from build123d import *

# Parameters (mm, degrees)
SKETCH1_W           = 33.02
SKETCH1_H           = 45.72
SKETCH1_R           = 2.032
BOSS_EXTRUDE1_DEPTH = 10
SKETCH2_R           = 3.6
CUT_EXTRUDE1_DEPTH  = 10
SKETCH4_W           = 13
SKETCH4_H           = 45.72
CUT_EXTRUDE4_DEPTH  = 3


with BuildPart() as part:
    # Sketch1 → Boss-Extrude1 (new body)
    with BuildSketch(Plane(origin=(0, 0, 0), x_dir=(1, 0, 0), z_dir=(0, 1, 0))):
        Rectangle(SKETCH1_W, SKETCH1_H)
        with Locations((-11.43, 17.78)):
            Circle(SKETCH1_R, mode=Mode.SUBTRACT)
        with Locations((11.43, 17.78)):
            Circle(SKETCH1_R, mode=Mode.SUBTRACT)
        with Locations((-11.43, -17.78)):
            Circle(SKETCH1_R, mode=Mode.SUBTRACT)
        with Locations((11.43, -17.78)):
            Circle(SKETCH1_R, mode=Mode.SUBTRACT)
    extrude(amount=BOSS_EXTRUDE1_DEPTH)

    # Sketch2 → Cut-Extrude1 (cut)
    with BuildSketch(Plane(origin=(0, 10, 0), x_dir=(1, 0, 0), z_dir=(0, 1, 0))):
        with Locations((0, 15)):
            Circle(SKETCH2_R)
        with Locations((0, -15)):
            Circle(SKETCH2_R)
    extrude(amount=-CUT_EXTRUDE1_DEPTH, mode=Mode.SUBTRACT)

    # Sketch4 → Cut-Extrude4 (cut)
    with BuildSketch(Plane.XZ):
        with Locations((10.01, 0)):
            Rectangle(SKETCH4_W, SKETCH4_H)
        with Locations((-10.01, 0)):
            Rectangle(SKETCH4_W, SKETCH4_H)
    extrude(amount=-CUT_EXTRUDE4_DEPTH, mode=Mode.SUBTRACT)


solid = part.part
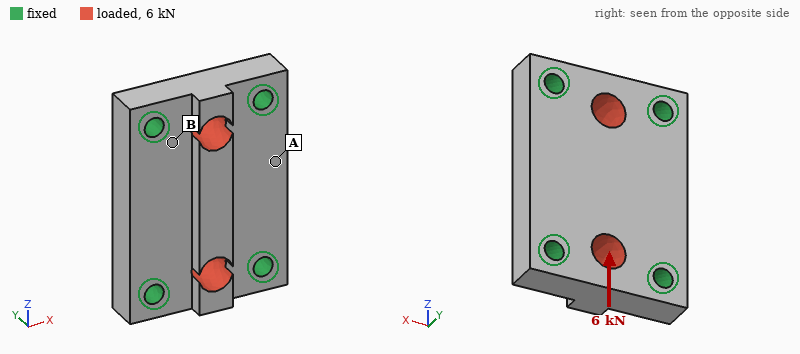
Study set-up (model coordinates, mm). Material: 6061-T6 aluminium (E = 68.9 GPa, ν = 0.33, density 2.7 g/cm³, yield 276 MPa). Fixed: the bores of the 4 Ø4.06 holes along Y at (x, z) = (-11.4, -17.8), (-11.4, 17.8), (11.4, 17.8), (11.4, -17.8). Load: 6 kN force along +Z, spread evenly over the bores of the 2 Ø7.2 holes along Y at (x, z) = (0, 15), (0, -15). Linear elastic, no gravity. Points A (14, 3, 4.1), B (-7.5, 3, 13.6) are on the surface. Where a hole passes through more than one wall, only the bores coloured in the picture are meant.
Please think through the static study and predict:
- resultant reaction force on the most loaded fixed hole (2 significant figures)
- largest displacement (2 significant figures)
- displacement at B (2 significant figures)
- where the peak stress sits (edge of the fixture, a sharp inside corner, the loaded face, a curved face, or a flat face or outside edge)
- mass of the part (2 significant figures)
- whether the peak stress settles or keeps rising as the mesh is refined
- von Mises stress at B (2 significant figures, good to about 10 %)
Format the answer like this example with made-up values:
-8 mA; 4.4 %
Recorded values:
1.5 kN; 14 µm; 2.5 µm; a sharp inside corner; 28 g; keeps rising; 27 MPa
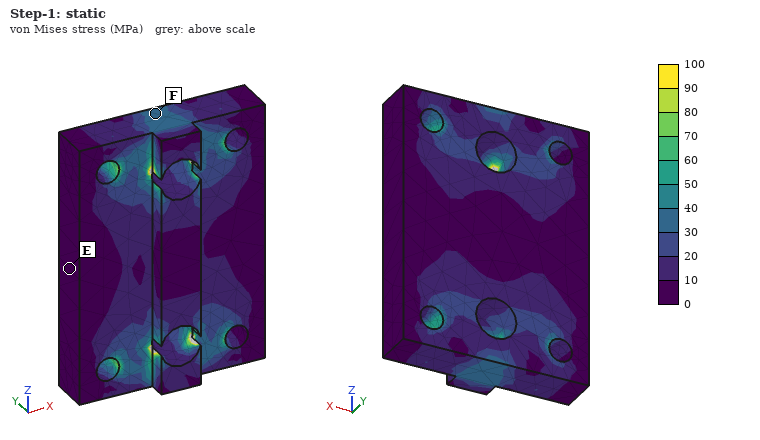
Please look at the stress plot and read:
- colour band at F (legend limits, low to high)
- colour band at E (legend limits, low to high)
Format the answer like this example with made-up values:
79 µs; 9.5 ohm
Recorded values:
30 to 40 MPa; 0 to 10 MPa
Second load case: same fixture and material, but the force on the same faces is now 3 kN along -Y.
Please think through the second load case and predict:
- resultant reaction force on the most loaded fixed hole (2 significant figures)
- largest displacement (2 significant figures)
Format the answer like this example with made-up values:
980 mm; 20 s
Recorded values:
750 N; 10 µm
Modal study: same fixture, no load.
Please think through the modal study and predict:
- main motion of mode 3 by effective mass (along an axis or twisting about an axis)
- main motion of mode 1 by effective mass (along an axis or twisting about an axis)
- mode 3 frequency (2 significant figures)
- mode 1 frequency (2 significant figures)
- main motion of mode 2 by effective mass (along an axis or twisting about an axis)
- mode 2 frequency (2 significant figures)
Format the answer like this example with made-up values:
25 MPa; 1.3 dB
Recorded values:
along X; along Y; 34 kHz; 22 kHz; twisting about Z; 29 kHz
